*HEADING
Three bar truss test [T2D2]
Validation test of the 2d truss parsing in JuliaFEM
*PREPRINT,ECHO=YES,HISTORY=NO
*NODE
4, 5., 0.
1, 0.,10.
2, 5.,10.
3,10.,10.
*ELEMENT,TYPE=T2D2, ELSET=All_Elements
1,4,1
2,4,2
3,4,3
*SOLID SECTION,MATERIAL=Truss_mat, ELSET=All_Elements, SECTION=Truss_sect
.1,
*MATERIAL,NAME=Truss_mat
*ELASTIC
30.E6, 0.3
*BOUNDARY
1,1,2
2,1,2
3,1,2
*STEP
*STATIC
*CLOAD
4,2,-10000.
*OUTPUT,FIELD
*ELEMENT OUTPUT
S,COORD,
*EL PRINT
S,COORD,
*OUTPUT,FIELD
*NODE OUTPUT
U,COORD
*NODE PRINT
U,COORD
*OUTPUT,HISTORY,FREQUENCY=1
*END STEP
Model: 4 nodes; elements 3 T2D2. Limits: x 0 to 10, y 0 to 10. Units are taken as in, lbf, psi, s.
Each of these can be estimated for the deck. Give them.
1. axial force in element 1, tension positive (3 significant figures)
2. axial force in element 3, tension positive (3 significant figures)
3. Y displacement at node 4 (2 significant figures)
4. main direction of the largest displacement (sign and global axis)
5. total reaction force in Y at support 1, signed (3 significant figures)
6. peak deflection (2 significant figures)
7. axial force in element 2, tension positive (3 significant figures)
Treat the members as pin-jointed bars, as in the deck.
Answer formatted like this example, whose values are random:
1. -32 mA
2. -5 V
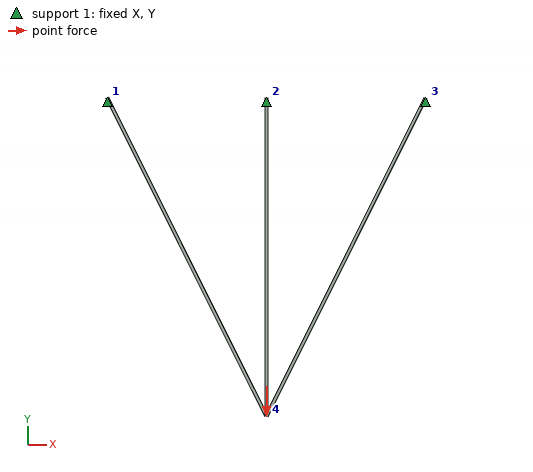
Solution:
1. 3290 lbf
2. 3290 lbf
3. -0.014 in
4. -Y
5. 10000 lbf
6. 0.014 in
7. 4110 lbf
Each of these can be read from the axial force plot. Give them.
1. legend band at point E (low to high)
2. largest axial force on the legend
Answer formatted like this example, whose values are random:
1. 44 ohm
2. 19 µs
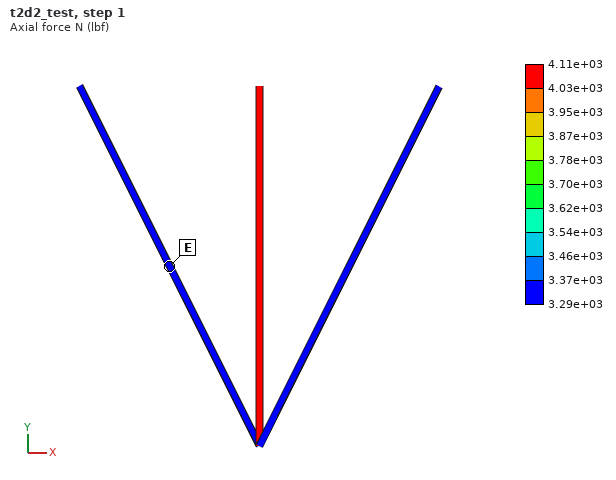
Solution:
1. 3.29e+03 to 3.37e+03 lbf
2. 4.11e+03 lbf
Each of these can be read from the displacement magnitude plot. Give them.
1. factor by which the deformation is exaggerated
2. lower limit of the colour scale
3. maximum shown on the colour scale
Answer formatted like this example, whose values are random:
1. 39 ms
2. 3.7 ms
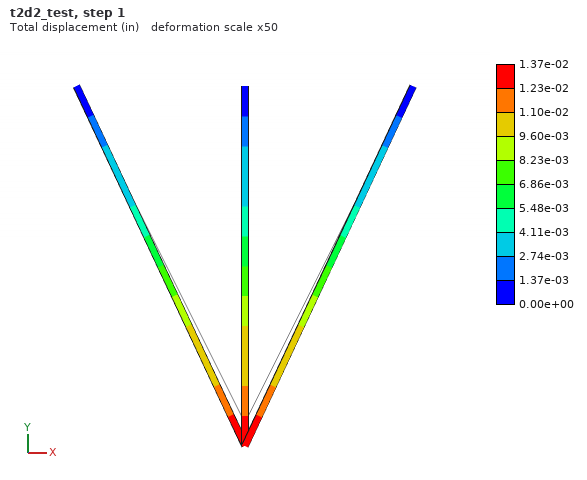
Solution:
1. 50
2. 0.00e+00 in
3. 1.37e-02 in
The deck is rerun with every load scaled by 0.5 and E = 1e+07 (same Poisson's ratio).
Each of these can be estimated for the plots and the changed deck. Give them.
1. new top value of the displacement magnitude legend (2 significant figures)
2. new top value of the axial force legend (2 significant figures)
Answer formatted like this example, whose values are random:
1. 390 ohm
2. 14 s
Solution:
1. 0.021 in
2. 2100 lbf
